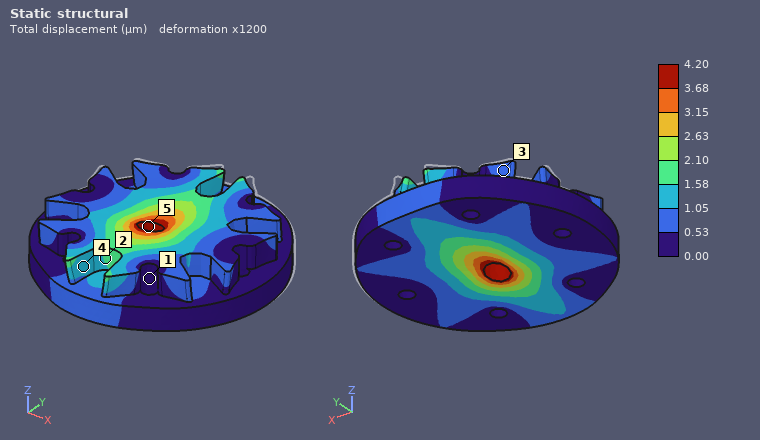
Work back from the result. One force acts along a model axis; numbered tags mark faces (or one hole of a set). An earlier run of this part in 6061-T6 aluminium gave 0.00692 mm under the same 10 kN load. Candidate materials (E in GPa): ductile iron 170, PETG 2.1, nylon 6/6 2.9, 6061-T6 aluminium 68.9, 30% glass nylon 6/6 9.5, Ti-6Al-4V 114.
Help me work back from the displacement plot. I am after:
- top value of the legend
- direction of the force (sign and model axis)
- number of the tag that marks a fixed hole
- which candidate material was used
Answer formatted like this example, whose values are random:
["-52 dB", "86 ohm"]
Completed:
["4.20 µm", "-Y", "1", "Ti-6Al-4V"]
